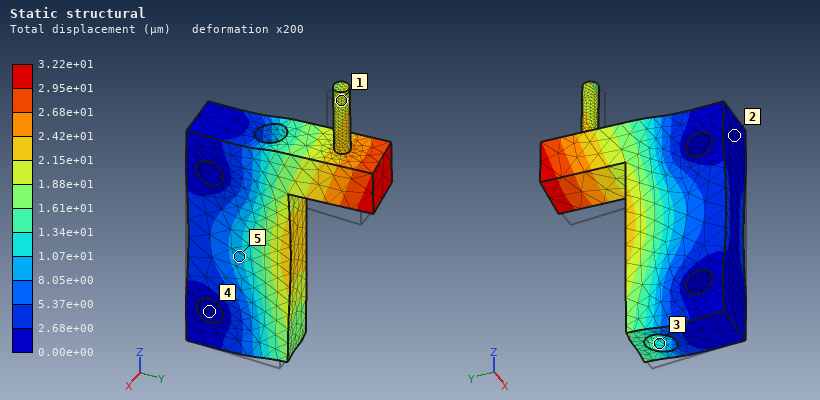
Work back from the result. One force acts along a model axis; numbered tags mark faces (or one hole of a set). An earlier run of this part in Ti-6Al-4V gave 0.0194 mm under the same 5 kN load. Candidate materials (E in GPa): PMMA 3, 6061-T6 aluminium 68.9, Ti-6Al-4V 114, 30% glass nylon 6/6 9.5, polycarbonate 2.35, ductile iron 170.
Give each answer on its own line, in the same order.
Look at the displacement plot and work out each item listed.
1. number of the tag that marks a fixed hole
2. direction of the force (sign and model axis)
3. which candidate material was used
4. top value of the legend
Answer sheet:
4
-X
6061-T6 aluminium
3.22e+01 µm
